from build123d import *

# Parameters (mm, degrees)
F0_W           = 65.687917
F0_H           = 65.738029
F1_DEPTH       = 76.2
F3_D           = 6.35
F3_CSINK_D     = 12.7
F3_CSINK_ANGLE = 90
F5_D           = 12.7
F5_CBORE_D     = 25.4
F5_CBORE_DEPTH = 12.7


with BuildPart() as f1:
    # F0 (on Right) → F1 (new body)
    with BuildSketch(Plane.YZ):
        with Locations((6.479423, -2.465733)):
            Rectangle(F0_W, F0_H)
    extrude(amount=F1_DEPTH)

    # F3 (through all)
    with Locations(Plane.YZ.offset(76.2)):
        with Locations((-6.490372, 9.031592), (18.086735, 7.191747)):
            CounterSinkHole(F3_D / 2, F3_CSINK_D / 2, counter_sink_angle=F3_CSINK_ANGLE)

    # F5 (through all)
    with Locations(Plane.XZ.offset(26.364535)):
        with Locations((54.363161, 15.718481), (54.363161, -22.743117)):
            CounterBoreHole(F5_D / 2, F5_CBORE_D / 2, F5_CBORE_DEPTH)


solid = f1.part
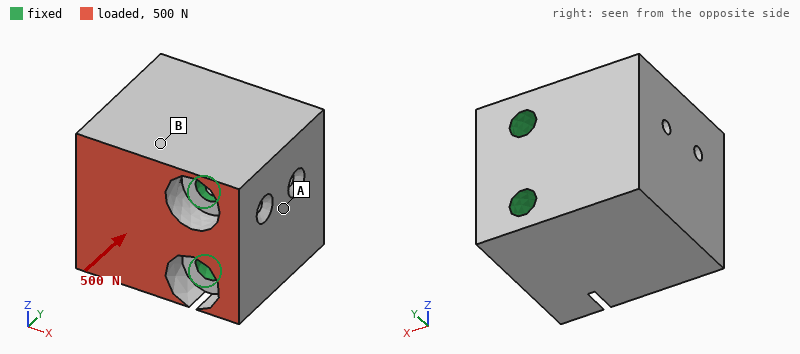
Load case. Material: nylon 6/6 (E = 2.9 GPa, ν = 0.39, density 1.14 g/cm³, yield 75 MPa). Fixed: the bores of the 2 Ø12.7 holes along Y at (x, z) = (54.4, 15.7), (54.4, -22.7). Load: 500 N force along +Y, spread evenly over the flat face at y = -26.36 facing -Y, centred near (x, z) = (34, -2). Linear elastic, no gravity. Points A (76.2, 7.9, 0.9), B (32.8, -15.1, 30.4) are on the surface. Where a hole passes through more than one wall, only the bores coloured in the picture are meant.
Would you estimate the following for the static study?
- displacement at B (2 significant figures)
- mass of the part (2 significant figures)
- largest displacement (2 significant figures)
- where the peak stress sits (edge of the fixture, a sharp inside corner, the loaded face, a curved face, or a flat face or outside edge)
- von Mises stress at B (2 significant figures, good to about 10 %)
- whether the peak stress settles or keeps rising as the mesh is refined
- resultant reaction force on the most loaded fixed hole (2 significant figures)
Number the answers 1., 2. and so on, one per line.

1. 4.3 µm
2. 340 g
3. 9.3 µm
4. edge of the fixture
5. 0.17 MPa
6. keeps rising
7. 250 N
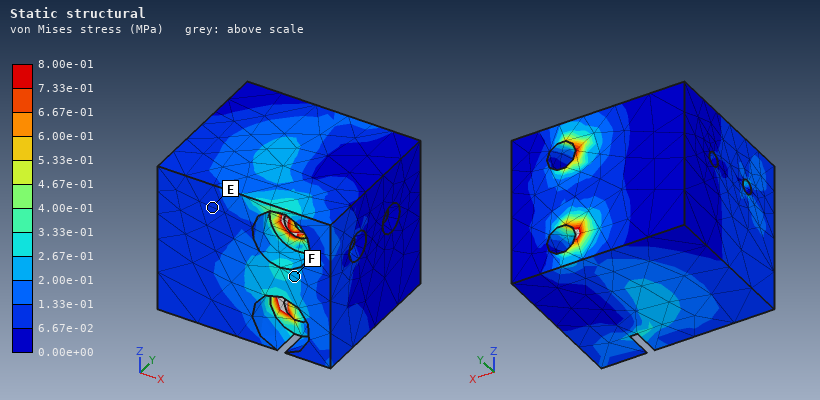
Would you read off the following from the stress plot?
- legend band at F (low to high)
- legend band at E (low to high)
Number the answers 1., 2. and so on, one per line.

1. 2.00e-01 to 2.67e-01 MPa
2. 6.67e-02 to 1.33e-01 MPa
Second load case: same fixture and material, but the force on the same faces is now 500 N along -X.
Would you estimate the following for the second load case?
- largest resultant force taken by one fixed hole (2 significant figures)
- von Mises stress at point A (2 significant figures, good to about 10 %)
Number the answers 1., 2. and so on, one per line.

1. 260 N
2. 0.18 MPa
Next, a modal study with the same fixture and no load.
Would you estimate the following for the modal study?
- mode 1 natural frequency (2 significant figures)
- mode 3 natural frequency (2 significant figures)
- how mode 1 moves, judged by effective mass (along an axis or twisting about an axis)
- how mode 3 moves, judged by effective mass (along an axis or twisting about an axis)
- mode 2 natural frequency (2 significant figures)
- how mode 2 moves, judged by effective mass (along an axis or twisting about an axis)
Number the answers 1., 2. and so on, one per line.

1. 2800 Hz
2. 3900 Hz
3. along Y
4. twisting about X
5. 3100 Hz
6. along Z
